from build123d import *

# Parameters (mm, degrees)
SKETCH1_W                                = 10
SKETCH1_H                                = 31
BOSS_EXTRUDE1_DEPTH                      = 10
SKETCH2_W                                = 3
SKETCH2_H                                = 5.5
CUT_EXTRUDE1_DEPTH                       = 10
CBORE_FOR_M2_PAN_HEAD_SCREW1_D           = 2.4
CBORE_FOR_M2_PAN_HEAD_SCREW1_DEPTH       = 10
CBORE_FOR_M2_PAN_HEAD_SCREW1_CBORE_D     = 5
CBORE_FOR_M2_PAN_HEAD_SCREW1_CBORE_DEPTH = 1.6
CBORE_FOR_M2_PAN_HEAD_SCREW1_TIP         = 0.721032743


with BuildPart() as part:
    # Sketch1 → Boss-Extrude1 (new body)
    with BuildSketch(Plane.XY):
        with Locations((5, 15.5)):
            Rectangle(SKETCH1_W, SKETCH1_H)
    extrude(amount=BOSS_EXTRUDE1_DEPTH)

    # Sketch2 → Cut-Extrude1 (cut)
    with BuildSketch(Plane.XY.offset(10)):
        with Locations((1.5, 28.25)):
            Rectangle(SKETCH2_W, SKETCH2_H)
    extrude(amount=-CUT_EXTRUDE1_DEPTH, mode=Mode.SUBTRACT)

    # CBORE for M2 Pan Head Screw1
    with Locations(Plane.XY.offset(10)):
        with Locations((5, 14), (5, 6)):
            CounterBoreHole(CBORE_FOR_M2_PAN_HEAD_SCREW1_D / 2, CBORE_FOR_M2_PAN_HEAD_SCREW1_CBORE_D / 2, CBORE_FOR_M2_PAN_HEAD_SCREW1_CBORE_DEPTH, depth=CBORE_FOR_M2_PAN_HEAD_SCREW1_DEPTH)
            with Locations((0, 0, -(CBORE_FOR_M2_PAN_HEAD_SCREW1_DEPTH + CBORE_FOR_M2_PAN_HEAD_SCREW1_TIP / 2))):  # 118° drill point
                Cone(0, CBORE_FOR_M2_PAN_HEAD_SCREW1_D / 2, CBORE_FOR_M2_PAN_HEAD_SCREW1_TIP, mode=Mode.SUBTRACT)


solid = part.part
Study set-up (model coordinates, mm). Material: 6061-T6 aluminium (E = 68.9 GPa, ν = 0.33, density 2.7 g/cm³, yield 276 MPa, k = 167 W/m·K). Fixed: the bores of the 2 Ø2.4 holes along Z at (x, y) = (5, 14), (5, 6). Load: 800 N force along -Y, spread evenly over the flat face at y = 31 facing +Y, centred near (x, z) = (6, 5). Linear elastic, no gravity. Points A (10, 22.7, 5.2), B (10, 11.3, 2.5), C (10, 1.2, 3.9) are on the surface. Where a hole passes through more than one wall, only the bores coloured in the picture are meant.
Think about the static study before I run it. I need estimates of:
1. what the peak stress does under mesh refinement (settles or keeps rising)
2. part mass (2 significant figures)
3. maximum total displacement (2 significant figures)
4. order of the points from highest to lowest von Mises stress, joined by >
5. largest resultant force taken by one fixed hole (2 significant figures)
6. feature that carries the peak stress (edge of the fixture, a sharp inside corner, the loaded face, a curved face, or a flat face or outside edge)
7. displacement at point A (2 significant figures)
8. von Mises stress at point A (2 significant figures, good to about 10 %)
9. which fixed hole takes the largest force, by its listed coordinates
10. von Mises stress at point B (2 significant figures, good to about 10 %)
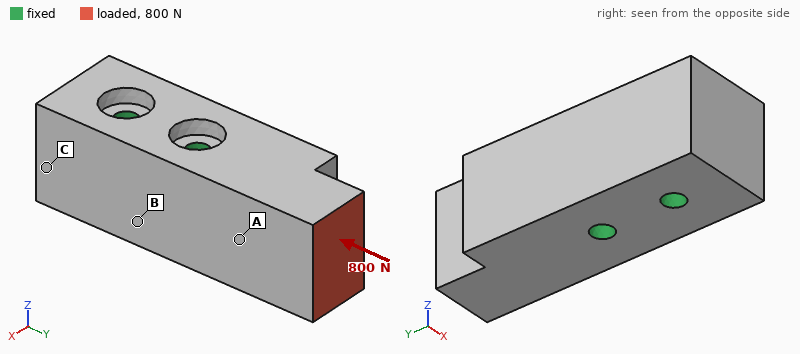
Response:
keeps rising
7.5 g
6.1 µm
A > B > C
660 N
edge of the fixture
3.2 µm
14 MPa
(5, 14)
7.3 MPa
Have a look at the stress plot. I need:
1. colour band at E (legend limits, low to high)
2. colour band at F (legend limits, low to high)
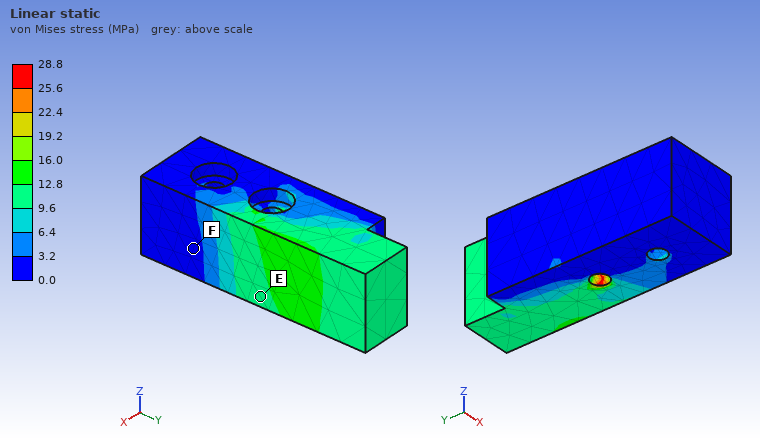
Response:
9.6 to 12.8 MPa
0.0 to 3.2 MPa
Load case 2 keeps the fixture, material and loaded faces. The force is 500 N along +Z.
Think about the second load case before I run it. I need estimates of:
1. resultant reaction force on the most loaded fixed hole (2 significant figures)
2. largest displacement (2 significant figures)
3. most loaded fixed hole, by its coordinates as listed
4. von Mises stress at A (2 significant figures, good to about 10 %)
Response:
730 N
28 µm
(5, 14)
17 MPa
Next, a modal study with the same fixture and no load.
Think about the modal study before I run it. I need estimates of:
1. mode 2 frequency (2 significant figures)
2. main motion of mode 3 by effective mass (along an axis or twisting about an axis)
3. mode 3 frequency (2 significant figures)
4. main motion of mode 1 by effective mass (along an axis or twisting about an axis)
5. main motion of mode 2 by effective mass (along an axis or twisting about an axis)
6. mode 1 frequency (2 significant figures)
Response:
22 kHz
twisting about Y
43 kHz
along X
along Z
20 kHz
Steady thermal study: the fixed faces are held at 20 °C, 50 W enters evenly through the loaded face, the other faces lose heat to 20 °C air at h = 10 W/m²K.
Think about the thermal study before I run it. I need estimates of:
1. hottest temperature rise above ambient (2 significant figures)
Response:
63 K
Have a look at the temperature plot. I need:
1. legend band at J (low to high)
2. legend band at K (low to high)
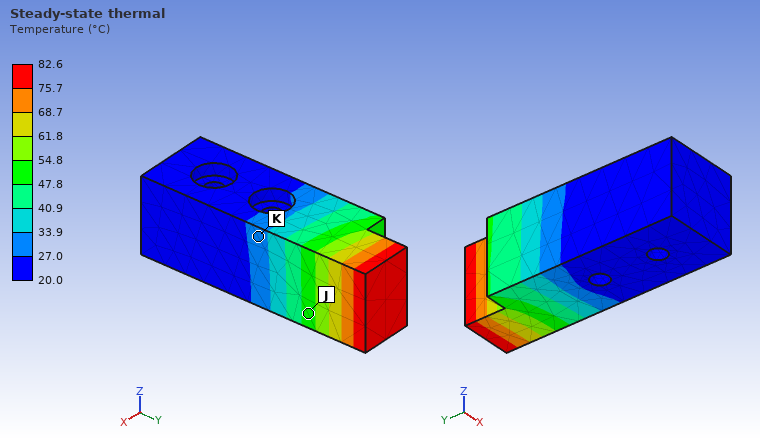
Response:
47.8 to 54.8 °C
27.0 to 33.9 °C
